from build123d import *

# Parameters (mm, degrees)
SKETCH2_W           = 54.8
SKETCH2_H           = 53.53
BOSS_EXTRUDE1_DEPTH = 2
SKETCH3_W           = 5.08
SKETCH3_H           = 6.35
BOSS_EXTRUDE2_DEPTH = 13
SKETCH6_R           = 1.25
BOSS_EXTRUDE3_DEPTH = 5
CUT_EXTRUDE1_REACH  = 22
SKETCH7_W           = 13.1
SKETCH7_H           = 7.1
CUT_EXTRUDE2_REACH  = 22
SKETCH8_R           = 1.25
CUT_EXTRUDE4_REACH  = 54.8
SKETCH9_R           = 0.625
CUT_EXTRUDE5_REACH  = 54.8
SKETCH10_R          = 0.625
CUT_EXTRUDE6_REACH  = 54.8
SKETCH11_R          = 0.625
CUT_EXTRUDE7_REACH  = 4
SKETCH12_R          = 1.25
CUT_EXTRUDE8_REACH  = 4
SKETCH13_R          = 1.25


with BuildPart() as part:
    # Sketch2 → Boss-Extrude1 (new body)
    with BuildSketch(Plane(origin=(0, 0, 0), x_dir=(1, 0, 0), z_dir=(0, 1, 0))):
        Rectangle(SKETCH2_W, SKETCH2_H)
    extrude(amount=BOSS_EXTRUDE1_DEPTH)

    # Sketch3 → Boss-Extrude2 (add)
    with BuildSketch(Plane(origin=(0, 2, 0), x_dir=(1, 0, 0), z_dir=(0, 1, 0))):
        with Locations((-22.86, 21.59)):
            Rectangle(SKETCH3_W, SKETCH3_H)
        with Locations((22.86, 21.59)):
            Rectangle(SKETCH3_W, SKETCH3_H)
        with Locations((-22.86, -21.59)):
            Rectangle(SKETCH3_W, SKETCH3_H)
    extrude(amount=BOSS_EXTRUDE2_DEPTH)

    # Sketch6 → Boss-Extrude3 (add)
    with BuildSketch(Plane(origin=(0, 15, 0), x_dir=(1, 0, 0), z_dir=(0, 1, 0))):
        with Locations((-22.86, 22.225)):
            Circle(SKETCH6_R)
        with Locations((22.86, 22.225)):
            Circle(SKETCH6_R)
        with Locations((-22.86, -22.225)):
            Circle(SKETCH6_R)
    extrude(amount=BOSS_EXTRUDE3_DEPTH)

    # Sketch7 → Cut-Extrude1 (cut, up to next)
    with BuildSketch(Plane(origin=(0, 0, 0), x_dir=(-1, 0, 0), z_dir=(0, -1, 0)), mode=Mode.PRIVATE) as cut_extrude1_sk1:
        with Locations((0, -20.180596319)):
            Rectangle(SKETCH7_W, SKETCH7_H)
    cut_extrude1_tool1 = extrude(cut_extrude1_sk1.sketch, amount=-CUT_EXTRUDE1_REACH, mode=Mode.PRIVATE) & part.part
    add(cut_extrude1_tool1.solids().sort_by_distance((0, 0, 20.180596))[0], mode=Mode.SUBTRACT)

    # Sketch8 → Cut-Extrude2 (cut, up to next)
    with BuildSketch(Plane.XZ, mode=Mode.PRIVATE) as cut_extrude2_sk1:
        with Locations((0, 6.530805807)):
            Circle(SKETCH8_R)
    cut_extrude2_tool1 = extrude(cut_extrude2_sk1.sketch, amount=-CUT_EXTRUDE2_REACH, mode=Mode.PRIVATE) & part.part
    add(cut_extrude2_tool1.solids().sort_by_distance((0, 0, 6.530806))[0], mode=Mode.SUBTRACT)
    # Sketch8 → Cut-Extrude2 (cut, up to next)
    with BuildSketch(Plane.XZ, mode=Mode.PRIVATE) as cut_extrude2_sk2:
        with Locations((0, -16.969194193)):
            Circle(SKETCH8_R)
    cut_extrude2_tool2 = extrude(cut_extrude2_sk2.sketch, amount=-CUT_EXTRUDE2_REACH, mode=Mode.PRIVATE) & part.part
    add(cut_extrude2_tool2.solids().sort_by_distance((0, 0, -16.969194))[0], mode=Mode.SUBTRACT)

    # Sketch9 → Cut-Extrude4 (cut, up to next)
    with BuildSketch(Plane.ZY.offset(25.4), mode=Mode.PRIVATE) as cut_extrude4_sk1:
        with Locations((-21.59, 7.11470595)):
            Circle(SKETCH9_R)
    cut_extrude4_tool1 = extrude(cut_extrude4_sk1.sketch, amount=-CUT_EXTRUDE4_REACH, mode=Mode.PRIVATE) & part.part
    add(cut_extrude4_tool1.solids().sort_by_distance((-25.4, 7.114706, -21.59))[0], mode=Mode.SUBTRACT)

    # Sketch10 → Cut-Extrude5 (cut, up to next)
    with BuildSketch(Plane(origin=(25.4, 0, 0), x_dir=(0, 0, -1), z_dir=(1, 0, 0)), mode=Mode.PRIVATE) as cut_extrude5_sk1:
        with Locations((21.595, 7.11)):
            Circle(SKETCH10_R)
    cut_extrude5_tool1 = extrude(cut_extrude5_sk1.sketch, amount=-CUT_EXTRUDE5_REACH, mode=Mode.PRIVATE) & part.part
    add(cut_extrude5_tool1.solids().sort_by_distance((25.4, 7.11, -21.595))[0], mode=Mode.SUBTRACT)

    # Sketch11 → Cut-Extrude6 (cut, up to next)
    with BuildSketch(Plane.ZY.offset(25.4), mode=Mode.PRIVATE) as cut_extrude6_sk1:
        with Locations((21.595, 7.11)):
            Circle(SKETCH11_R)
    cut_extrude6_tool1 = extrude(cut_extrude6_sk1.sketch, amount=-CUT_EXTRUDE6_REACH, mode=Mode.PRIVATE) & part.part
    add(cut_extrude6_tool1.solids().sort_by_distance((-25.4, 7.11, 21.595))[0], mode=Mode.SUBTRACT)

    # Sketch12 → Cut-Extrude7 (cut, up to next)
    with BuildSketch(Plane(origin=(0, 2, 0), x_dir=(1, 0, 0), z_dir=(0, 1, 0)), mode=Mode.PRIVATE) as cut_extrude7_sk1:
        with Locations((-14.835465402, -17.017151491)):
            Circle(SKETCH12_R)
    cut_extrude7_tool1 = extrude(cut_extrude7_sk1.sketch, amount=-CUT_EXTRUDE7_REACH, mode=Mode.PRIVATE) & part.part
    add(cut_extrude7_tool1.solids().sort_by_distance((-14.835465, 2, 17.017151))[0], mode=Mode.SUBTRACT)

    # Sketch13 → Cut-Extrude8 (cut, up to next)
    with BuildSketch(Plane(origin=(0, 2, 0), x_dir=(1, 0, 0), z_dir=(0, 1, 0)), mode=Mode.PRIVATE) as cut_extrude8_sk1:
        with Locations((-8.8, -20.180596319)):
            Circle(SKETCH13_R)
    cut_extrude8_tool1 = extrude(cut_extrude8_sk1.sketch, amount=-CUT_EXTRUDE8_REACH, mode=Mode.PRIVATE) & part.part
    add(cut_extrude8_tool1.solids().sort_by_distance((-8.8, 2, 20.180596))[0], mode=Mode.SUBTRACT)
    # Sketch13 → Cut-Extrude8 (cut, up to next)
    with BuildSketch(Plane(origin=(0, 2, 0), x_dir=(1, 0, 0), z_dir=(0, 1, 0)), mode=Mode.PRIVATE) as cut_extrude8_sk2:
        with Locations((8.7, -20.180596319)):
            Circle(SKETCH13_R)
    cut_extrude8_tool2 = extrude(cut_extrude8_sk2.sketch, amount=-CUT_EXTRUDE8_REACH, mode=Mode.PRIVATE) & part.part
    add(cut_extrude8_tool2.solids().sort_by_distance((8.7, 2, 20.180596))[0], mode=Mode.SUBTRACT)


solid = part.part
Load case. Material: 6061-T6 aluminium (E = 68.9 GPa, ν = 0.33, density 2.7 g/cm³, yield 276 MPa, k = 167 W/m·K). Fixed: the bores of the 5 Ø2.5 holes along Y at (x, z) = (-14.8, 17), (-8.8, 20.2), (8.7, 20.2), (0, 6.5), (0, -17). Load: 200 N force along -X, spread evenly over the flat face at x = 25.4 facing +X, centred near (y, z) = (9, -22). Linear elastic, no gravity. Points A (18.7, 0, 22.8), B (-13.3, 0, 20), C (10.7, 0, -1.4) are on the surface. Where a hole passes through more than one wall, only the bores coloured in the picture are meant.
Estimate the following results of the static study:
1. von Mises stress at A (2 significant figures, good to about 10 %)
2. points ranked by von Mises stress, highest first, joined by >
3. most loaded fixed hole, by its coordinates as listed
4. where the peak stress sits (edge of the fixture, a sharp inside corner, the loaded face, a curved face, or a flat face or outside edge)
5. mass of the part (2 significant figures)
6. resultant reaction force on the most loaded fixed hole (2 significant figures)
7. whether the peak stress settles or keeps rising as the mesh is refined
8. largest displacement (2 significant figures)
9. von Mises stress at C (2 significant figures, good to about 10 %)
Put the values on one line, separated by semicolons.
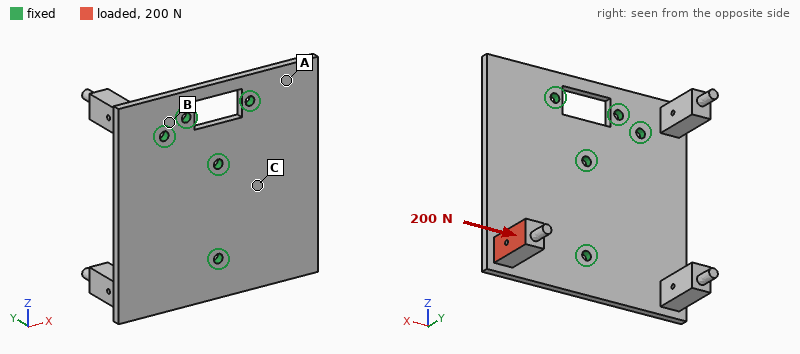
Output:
21 MPa; C > A > B; (0, -17); edge of the fixture; 19 g; 200 N; keeps rising; 0.57 mm; 38 MPa
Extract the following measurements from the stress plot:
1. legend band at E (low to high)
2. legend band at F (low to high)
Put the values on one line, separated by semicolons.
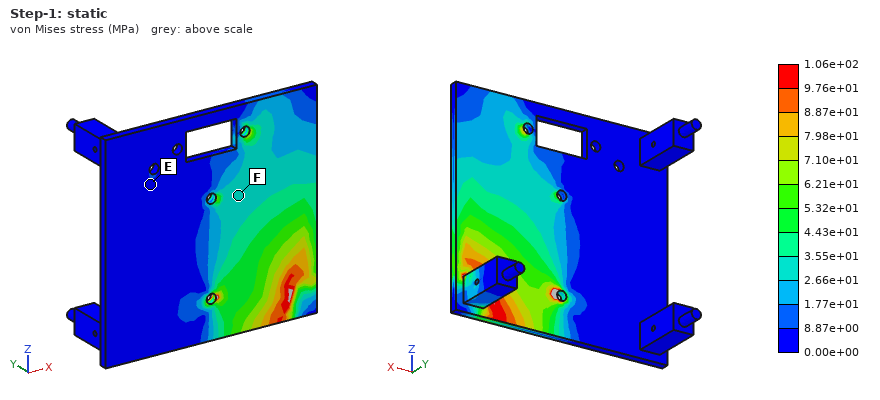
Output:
0.00e+00 to 8.87e+00 MPa; 2.66e+01 to 3.55e+01 MPa
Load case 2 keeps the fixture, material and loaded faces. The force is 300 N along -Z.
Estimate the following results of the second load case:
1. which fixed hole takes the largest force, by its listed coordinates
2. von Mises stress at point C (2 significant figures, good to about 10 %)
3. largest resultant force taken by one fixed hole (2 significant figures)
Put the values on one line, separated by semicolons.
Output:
(0, -17); 16 MPa; 210 N
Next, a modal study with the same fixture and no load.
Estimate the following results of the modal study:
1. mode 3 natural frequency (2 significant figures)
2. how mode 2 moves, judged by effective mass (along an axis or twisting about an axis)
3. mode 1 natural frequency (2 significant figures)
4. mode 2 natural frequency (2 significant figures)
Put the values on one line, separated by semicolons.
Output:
3500 Hz; along Y; 1700 Hz; 1900 Hz
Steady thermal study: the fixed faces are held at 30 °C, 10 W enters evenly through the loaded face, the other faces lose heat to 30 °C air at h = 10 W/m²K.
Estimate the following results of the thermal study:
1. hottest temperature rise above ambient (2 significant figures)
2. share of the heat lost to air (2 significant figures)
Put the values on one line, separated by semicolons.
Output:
44 K; 4.1 %
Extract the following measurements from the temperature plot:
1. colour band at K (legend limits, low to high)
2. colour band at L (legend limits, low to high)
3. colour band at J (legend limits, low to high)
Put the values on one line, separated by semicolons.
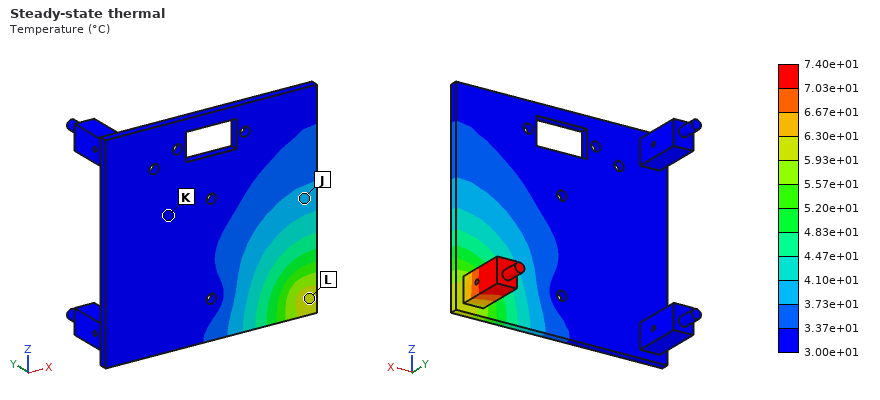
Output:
3.00e+01 to 3.37e+01 °C; 5.93e+01 to 6.30e+01 °C; 3.73e+01 to 4.10e+01 °C
